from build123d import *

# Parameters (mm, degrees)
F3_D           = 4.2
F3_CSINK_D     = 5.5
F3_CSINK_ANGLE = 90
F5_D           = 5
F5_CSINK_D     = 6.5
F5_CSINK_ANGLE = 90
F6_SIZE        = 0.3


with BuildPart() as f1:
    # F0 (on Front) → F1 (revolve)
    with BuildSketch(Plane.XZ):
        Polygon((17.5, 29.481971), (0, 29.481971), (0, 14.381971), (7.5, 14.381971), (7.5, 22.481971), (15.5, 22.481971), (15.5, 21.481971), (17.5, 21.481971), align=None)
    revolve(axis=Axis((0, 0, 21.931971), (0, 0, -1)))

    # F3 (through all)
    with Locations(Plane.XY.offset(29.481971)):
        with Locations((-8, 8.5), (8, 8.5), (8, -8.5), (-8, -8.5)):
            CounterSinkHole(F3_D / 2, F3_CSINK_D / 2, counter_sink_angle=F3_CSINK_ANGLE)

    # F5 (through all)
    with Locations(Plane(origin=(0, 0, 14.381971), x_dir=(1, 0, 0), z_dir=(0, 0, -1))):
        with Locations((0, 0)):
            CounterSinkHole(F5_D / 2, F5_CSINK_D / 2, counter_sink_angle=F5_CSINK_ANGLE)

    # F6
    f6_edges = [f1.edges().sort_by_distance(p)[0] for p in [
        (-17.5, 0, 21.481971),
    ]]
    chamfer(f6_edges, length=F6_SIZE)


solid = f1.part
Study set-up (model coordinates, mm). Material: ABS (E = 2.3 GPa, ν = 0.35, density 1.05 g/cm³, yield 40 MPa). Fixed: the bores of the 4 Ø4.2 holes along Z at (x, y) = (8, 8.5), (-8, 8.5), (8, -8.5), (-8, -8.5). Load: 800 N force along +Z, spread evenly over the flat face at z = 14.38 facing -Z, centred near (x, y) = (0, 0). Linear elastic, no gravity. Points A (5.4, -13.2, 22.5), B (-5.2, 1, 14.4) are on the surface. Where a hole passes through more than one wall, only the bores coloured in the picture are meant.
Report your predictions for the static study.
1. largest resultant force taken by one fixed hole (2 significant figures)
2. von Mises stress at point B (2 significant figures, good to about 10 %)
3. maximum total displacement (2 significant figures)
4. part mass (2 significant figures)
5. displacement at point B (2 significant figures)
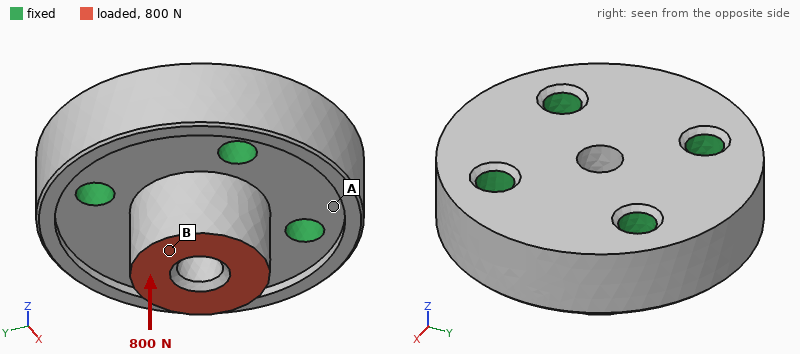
210 N
5.5 MPa
43 µm
8.1 g
40 µm
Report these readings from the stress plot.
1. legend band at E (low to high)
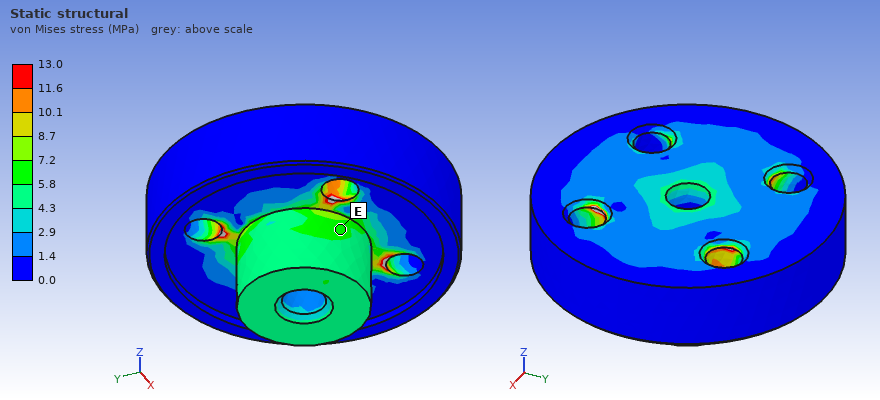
5.8 to 7.2 MPa
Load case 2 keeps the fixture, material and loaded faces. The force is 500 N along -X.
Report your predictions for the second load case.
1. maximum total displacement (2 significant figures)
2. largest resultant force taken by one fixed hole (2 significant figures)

0.12 mm
220 N
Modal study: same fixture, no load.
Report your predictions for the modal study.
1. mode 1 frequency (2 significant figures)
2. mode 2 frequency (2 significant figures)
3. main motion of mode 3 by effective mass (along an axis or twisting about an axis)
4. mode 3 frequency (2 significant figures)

13 kHz
14 kHz
along Z
15 kHz
